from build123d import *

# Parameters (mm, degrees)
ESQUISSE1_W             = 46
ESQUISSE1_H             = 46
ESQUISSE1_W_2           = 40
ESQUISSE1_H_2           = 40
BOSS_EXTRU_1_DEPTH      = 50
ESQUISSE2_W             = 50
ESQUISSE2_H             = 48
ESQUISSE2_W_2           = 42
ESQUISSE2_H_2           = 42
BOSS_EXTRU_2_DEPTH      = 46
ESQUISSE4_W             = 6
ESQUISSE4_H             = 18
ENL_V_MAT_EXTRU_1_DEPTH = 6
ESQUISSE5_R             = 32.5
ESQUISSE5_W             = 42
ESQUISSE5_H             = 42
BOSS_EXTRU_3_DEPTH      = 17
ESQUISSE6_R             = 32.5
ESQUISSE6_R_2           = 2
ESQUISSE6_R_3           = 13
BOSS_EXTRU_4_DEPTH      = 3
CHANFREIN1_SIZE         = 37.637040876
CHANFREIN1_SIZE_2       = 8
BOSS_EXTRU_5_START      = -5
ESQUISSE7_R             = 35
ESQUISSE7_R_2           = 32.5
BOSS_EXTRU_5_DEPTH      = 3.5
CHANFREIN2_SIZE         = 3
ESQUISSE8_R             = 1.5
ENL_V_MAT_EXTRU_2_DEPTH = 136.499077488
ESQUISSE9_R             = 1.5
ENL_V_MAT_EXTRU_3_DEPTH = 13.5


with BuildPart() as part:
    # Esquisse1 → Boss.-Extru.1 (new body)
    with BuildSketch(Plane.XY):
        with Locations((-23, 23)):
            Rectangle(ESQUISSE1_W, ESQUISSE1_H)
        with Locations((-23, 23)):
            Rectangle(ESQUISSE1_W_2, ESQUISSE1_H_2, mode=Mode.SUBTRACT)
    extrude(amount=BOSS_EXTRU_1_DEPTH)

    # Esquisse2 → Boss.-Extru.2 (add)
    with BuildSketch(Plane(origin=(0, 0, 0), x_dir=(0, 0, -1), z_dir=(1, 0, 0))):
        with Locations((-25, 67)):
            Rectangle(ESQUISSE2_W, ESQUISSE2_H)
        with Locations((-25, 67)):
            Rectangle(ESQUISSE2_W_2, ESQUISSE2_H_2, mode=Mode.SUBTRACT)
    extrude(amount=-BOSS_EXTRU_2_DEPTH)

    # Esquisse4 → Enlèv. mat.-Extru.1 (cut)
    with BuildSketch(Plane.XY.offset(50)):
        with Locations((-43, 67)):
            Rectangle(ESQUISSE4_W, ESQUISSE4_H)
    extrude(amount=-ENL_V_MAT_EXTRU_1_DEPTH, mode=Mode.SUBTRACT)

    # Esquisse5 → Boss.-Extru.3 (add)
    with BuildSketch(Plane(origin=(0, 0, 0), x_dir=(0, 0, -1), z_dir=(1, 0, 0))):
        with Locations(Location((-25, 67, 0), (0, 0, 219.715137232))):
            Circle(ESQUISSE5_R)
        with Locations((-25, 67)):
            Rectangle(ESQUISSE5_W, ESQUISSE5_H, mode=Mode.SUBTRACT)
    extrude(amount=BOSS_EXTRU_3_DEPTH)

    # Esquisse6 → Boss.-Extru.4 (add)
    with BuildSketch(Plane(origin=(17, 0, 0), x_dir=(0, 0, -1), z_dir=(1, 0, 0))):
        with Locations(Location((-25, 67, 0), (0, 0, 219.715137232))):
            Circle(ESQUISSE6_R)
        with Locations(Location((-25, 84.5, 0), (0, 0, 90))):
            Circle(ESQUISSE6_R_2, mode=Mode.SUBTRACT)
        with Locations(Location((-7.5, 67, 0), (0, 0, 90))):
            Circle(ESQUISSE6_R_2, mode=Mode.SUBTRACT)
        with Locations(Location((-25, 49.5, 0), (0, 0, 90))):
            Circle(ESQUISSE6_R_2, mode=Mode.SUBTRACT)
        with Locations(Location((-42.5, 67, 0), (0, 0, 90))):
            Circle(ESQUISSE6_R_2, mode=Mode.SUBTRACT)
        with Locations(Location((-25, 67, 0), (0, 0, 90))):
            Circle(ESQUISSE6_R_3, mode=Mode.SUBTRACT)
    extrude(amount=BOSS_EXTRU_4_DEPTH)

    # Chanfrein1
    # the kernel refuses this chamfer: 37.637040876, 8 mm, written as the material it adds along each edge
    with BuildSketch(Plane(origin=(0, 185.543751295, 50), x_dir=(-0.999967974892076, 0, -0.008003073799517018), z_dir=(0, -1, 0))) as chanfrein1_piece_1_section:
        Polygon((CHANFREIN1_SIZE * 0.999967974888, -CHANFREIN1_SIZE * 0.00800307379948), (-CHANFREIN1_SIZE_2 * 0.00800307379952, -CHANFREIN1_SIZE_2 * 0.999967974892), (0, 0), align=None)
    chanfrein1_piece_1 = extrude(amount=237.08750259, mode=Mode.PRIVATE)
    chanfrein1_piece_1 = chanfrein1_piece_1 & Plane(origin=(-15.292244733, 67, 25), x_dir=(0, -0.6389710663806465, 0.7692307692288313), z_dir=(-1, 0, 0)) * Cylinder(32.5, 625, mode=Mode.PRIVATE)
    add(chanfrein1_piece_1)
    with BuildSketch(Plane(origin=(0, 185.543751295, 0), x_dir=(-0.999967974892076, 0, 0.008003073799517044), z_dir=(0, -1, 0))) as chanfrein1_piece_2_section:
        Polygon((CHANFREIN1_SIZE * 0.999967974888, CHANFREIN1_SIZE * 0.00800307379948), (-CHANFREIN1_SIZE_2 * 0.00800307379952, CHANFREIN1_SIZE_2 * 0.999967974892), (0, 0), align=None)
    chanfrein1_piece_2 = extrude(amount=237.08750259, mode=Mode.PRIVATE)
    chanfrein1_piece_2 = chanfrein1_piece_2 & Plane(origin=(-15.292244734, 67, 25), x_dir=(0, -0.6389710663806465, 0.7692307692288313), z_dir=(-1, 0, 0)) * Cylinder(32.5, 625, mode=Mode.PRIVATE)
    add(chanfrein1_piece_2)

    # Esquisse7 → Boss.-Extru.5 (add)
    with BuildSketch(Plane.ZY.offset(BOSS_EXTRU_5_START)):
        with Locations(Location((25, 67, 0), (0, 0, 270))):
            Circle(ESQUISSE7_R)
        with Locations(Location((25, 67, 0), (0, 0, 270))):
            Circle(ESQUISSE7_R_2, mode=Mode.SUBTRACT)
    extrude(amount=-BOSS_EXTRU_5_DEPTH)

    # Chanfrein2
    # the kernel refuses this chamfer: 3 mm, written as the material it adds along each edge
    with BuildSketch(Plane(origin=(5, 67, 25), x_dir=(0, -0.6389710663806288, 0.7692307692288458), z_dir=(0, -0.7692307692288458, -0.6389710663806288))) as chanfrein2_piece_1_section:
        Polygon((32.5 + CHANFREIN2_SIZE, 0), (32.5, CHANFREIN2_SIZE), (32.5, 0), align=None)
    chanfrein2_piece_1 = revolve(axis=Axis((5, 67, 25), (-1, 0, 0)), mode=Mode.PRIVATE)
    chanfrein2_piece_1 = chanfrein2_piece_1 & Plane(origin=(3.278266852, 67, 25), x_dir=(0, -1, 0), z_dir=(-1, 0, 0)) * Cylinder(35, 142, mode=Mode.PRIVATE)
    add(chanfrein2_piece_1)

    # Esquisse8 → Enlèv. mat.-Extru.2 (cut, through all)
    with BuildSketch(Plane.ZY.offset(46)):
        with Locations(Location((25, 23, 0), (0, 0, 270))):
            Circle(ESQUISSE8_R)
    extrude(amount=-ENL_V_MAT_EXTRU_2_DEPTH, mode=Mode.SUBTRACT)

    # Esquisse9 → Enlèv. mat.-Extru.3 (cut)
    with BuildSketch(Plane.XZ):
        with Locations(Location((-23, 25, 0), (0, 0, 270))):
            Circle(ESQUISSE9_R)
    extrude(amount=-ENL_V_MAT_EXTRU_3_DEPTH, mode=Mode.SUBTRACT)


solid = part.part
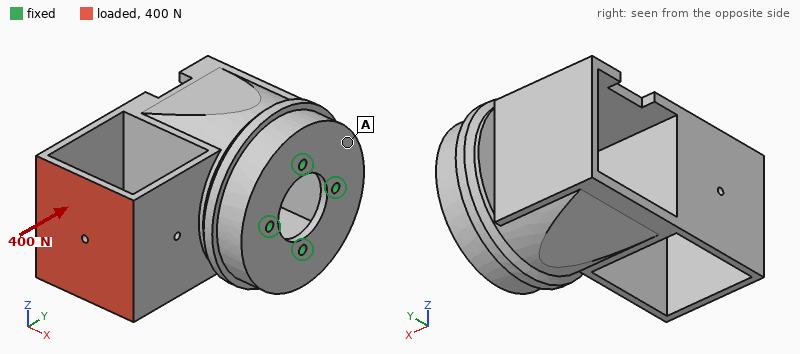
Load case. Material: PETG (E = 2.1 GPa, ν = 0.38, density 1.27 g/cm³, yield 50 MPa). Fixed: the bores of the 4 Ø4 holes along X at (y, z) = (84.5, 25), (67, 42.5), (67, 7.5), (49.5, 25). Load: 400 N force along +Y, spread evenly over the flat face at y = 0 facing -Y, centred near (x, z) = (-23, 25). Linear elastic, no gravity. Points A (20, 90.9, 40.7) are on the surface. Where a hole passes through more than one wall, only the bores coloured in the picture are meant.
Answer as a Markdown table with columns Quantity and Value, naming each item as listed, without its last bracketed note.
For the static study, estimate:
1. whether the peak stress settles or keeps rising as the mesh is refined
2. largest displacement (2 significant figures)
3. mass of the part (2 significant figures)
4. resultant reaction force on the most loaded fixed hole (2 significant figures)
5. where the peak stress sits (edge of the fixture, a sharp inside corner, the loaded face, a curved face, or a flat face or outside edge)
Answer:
| Quantity | Value |
|---|---|
| whether the peak stress settles or keeps rising as the mesh is refined | keeps rising |
| largest displacement | 1.4 mm |
| mass of the part | 120 g |
| resultant reaction force on the most loaded fixed hole | 390 N |
| where the peak stress sits | edge of the fixture |
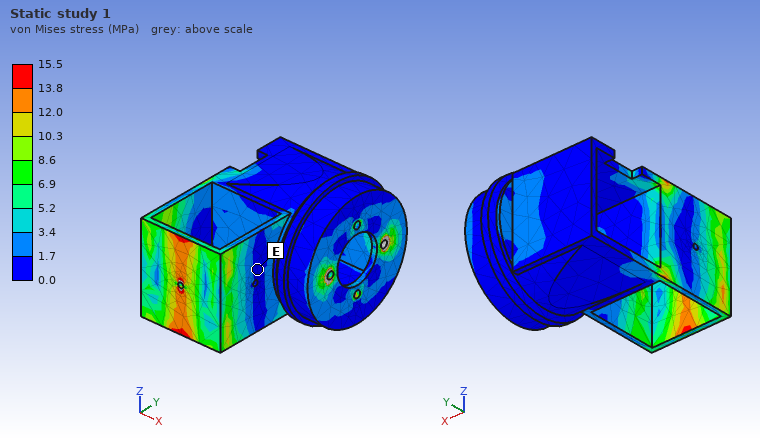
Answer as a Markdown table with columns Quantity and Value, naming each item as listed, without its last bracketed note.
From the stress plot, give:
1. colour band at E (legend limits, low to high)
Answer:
| Quantity | Value |
|---|---|
| colour band at E | 0.0 to 1.7 MPa |
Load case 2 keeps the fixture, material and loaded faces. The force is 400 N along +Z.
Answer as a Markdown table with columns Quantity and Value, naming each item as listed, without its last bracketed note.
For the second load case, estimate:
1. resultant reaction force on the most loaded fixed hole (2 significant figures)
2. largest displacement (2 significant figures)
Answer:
| Quantity | Value |
|---|---|
| resultant reaction force on the most loaded fixed hole | 560 N |
| largest displacement | 1.5 mm |
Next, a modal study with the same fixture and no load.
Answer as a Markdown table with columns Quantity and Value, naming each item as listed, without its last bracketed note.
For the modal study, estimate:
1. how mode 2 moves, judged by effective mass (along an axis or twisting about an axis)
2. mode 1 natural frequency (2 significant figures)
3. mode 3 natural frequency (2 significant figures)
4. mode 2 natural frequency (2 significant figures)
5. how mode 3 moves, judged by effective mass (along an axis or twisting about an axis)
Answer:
| Quantity | Value |
|---|---|
| how mode 2 moves, judged by effective mass | along Z |
| mode 1 natural frequency | 330 Hz |
| mode 3 natural frequency | 590 Hz |
| mode 2 natural frequency | 510 Hz |
| how mode 3 moves, judged by effective mass | along Y |
